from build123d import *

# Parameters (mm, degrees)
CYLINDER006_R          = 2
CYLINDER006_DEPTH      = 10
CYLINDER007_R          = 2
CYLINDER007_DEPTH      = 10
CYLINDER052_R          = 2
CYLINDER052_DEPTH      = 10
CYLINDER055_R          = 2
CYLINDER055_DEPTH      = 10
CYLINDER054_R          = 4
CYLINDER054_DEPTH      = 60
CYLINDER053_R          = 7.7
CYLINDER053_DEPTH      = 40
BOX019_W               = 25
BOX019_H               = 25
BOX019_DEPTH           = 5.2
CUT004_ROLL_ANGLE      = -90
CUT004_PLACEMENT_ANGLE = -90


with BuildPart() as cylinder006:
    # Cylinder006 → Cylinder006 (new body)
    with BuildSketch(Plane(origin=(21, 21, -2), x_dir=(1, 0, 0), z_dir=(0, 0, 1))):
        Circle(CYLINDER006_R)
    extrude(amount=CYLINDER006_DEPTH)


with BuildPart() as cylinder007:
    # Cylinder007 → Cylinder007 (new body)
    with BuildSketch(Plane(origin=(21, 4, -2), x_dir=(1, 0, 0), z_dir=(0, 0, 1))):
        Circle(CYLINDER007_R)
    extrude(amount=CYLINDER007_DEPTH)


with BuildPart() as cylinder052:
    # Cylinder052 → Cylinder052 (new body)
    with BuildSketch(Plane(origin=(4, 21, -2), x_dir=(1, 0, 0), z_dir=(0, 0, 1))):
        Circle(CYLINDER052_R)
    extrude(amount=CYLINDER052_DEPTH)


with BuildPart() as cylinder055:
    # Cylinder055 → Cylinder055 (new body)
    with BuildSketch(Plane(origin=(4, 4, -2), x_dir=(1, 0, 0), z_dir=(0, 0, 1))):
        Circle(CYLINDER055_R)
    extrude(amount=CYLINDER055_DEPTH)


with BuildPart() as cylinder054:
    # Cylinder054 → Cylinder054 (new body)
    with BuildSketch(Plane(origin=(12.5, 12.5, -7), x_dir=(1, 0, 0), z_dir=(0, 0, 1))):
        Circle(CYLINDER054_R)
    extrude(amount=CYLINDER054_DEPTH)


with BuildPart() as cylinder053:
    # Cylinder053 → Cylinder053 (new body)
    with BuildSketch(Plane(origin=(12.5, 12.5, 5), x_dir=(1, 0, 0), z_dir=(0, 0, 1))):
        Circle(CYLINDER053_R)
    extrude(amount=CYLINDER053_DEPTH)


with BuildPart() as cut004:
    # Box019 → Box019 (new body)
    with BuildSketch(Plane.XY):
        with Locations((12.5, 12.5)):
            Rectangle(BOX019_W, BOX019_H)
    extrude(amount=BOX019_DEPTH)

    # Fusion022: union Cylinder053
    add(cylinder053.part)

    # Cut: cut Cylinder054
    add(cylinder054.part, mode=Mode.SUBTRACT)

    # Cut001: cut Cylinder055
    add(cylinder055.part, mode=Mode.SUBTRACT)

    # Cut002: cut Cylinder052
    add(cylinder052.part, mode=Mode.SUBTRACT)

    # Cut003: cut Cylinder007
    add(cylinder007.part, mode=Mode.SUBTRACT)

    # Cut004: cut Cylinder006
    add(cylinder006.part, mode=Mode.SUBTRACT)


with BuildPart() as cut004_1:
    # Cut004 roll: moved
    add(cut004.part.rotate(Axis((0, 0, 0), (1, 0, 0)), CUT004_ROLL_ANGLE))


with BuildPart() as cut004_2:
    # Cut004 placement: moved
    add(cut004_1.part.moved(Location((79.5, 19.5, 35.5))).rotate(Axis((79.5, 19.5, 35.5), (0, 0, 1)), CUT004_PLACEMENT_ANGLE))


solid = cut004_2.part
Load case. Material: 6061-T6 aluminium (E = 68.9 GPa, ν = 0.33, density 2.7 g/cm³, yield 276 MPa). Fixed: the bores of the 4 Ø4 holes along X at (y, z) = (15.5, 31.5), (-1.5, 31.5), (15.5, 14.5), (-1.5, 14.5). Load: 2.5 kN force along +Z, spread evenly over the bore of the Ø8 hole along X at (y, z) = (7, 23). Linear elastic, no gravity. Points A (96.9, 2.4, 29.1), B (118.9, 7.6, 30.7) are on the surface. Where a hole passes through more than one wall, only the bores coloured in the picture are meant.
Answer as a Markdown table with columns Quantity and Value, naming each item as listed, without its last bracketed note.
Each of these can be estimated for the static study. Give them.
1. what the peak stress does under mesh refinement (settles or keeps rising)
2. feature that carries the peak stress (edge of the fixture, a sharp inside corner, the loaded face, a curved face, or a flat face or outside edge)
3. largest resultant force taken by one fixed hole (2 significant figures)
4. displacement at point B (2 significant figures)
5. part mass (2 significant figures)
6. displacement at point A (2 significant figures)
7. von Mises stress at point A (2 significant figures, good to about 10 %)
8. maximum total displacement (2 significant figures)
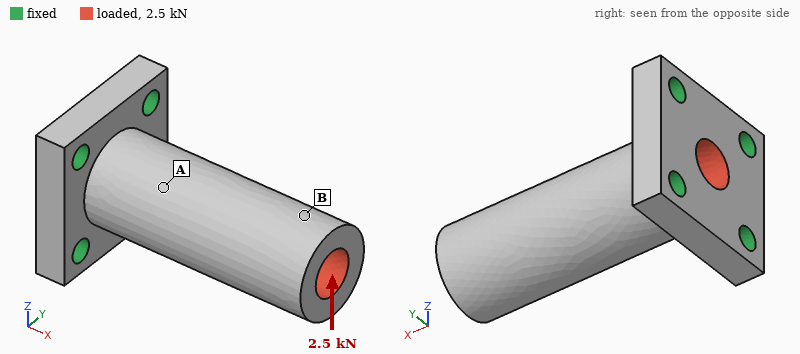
| Quantity | Value |
|---|---|
| what the peak stress does under mesh refinement | keeps rising |
| feature that carries the peak stress | edge of the fixture |
| largest resultant force taken by one fixed hole | 1.8 kN |
| displacement at point B | 0.16 mm |
| part mass | 22 g |
| displacement at point A | 0.053 mm |
| von Mises stress at point A | 53 MPa |
| maximum total displacement | 0.19 mm |
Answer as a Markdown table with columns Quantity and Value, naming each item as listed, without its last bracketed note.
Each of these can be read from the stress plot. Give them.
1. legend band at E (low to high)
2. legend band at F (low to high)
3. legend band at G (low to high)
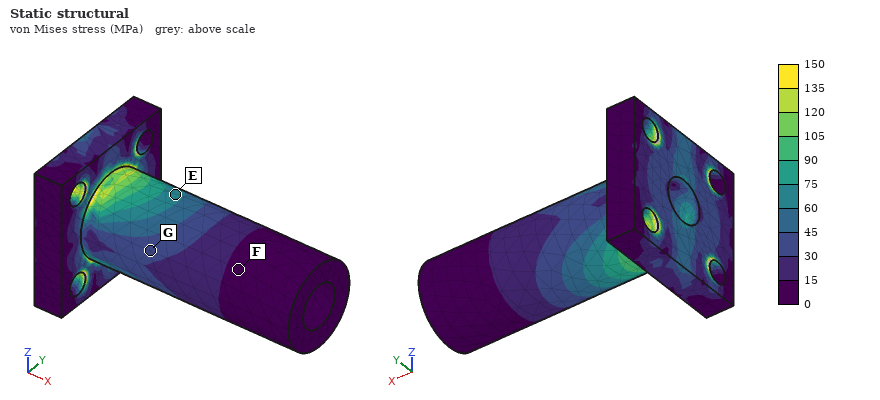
| Quantity | Value |
|---|---|
| legend band at E | 60 to 75 MPa |
| legend band at F | 0 to 15 MPa |
| legend band at G | 30 to 45 MPa |
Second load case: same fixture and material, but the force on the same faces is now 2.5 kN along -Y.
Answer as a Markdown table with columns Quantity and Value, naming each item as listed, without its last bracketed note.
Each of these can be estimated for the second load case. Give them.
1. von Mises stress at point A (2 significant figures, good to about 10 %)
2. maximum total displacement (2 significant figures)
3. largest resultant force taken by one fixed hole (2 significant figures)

| Quantity | Value |
|---|---|
| von Mises stress at point A | 44 MPa |
| maximum total displacement | 0.19 mm |
| largest resultant force taken by one fixed hole | 1.8 kN |
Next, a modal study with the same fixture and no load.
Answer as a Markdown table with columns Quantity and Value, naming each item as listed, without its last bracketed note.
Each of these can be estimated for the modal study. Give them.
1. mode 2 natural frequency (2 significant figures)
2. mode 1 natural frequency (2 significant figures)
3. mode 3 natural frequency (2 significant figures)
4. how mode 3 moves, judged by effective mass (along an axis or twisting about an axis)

| Quantity | Value |
|---|---|
| mode 2 natural frequency | 5500 Hz |
| mode 1 natural frequency | 5500 Hz |
| mode 3 natural frequency | 18 kHz |
| how mode 3 moves, judged by effective mass | twisting about X |
